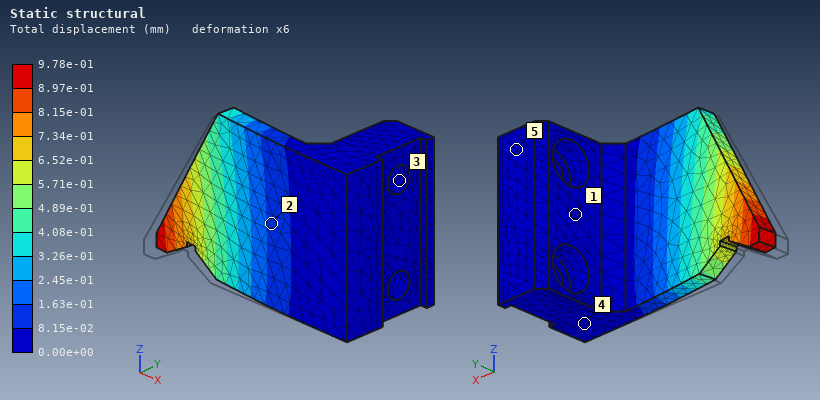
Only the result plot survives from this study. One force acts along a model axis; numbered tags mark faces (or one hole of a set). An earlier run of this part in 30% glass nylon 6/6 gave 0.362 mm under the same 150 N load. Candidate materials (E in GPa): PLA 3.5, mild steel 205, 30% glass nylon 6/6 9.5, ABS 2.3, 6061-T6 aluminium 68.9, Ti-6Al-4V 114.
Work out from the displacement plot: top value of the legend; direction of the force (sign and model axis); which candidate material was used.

9.78e-01 mm
+Y
PLA
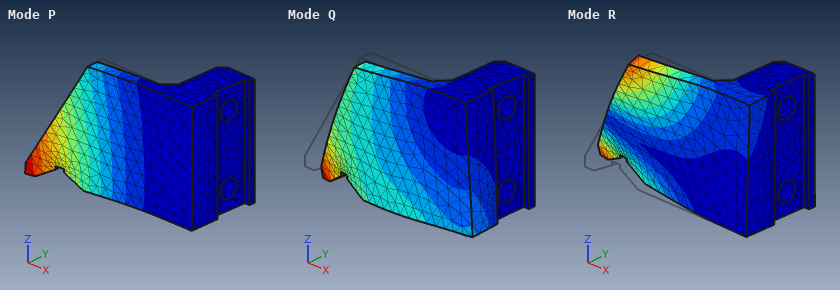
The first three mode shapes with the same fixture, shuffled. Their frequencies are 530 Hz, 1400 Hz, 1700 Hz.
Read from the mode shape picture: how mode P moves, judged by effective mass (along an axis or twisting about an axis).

along Y
